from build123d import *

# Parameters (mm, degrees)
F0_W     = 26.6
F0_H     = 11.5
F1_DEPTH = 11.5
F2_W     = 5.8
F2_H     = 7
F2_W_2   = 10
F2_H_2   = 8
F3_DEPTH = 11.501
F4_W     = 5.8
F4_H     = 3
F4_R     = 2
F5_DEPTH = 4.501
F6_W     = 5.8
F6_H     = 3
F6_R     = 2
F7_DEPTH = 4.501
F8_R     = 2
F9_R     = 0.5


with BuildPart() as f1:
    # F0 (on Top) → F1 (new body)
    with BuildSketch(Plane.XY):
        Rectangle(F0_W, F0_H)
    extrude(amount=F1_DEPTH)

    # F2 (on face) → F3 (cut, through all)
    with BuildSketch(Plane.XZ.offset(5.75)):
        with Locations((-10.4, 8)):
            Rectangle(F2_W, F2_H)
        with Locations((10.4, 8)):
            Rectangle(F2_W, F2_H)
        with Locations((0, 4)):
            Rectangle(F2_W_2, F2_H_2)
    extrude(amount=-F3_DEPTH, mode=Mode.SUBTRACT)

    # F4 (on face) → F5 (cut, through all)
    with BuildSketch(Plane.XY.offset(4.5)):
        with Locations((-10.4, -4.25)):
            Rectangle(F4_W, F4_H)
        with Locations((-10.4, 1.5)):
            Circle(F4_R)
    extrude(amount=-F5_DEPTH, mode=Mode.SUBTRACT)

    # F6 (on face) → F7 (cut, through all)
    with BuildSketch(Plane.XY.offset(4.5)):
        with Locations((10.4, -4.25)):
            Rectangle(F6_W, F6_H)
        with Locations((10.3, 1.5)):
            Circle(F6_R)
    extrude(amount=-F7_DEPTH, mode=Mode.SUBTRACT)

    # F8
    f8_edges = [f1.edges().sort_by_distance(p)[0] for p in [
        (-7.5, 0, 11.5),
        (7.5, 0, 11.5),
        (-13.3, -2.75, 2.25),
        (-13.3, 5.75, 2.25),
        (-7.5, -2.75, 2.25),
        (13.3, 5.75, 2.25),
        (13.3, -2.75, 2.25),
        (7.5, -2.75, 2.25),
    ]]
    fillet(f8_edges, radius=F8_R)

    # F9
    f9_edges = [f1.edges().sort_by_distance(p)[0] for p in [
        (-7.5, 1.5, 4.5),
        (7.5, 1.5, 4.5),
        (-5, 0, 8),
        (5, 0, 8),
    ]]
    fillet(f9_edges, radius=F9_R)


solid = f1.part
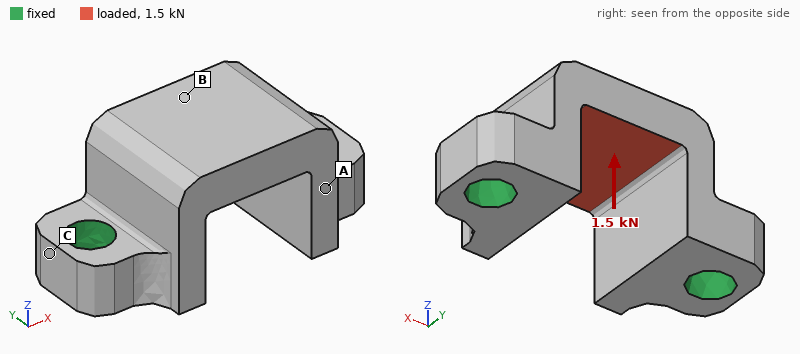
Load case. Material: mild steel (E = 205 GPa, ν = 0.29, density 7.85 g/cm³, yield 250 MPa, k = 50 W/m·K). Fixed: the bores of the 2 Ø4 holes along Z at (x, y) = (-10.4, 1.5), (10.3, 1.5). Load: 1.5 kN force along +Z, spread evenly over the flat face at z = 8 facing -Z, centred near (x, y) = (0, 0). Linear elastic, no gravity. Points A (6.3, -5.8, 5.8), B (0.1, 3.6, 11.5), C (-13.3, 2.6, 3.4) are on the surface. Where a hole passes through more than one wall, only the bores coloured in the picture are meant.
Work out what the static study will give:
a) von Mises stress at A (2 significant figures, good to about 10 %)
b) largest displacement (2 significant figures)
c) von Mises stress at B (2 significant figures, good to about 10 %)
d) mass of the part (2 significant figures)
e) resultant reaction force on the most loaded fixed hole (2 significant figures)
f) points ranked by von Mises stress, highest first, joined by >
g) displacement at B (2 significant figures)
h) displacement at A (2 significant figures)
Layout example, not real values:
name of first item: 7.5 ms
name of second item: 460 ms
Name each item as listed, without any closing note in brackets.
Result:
von Mises stress at A: 25 MPa
largest displacement: 6.5 µm
von Mises stress at B: 70 MPa
mass of the part: 11 g
resultant reaction force on the most loaded fixed hole: 830 N
points ranked by von Mises stress, highest first, joined by >: B > A > C
displacement at B: 4.1 µm
displacement at A: 2.9 µm
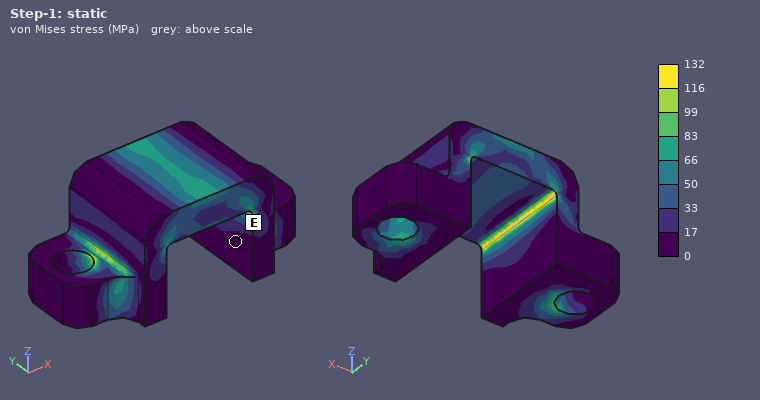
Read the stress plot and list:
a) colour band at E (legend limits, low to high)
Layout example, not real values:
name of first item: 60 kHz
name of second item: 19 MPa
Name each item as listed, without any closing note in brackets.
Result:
colour band at E: 0 to 17 MPa
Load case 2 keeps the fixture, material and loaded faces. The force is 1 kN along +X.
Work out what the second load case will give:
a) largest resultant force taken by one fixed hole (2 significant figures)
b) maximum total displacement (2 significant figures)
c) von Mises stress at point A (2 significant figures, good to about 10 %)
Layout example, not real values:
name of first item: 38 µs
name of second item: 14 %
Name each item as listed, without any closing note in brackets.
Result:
largest resultant force taken by one fixed hole: 520 N
maximum total displacement: 5.9 µm
von Mises stress at point A: 32 MPa
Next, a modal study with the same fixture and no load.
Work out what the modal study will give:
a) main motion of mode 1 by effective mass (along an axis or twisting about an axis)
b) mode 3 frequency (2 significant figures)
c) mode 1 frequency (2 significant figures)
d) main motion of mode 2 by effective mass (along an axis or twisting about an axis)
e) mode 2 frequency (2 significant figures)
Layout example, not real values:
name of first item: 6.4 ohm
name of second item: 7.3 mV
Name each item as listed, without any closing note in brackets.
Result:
main motion of mode 1 by effective mass: along Y
mode 3 frequency: 39 kHz
mode 1 frequency: 24 kHz
main motion of mode 2 by effective mass: along X
mode 2 frequency: 31 kHz
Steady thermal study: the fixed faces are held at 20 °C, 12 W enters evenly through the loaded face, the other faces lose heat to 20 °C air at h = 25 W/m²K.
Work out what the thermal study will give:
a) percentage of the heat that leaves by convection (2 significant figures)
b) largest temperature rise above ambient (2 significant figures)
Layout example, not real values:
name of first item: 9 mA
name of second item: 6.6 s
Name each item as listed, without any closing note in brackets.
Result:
percentage of the heat that leaves by convection: 3.7 %
largest temperature rise above ambient: 43 K
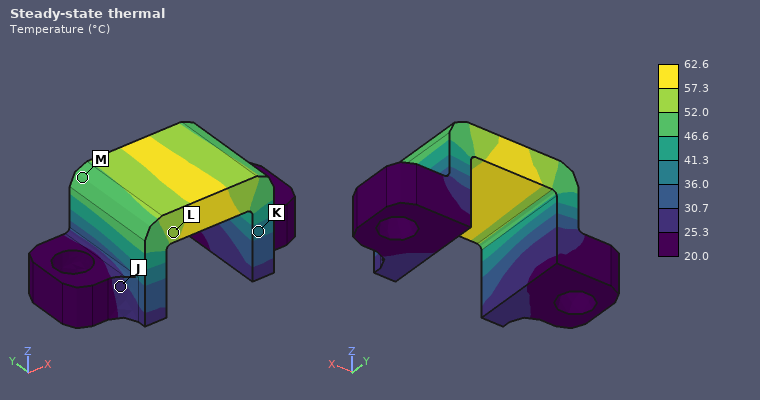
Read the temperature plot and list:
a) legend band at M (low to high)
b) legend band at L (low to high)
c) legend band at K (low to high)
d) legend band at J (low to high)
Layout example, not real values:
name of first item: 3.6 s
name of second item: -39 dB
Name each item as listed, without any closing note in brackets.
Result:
legend band at M: 46.6 to 52.0 °C
legend band at L: 52.0 to 57.3 °C
legend band at K: 36.0 to 41.3 °C
legend band at J: 25.3 to 30.7 °C
